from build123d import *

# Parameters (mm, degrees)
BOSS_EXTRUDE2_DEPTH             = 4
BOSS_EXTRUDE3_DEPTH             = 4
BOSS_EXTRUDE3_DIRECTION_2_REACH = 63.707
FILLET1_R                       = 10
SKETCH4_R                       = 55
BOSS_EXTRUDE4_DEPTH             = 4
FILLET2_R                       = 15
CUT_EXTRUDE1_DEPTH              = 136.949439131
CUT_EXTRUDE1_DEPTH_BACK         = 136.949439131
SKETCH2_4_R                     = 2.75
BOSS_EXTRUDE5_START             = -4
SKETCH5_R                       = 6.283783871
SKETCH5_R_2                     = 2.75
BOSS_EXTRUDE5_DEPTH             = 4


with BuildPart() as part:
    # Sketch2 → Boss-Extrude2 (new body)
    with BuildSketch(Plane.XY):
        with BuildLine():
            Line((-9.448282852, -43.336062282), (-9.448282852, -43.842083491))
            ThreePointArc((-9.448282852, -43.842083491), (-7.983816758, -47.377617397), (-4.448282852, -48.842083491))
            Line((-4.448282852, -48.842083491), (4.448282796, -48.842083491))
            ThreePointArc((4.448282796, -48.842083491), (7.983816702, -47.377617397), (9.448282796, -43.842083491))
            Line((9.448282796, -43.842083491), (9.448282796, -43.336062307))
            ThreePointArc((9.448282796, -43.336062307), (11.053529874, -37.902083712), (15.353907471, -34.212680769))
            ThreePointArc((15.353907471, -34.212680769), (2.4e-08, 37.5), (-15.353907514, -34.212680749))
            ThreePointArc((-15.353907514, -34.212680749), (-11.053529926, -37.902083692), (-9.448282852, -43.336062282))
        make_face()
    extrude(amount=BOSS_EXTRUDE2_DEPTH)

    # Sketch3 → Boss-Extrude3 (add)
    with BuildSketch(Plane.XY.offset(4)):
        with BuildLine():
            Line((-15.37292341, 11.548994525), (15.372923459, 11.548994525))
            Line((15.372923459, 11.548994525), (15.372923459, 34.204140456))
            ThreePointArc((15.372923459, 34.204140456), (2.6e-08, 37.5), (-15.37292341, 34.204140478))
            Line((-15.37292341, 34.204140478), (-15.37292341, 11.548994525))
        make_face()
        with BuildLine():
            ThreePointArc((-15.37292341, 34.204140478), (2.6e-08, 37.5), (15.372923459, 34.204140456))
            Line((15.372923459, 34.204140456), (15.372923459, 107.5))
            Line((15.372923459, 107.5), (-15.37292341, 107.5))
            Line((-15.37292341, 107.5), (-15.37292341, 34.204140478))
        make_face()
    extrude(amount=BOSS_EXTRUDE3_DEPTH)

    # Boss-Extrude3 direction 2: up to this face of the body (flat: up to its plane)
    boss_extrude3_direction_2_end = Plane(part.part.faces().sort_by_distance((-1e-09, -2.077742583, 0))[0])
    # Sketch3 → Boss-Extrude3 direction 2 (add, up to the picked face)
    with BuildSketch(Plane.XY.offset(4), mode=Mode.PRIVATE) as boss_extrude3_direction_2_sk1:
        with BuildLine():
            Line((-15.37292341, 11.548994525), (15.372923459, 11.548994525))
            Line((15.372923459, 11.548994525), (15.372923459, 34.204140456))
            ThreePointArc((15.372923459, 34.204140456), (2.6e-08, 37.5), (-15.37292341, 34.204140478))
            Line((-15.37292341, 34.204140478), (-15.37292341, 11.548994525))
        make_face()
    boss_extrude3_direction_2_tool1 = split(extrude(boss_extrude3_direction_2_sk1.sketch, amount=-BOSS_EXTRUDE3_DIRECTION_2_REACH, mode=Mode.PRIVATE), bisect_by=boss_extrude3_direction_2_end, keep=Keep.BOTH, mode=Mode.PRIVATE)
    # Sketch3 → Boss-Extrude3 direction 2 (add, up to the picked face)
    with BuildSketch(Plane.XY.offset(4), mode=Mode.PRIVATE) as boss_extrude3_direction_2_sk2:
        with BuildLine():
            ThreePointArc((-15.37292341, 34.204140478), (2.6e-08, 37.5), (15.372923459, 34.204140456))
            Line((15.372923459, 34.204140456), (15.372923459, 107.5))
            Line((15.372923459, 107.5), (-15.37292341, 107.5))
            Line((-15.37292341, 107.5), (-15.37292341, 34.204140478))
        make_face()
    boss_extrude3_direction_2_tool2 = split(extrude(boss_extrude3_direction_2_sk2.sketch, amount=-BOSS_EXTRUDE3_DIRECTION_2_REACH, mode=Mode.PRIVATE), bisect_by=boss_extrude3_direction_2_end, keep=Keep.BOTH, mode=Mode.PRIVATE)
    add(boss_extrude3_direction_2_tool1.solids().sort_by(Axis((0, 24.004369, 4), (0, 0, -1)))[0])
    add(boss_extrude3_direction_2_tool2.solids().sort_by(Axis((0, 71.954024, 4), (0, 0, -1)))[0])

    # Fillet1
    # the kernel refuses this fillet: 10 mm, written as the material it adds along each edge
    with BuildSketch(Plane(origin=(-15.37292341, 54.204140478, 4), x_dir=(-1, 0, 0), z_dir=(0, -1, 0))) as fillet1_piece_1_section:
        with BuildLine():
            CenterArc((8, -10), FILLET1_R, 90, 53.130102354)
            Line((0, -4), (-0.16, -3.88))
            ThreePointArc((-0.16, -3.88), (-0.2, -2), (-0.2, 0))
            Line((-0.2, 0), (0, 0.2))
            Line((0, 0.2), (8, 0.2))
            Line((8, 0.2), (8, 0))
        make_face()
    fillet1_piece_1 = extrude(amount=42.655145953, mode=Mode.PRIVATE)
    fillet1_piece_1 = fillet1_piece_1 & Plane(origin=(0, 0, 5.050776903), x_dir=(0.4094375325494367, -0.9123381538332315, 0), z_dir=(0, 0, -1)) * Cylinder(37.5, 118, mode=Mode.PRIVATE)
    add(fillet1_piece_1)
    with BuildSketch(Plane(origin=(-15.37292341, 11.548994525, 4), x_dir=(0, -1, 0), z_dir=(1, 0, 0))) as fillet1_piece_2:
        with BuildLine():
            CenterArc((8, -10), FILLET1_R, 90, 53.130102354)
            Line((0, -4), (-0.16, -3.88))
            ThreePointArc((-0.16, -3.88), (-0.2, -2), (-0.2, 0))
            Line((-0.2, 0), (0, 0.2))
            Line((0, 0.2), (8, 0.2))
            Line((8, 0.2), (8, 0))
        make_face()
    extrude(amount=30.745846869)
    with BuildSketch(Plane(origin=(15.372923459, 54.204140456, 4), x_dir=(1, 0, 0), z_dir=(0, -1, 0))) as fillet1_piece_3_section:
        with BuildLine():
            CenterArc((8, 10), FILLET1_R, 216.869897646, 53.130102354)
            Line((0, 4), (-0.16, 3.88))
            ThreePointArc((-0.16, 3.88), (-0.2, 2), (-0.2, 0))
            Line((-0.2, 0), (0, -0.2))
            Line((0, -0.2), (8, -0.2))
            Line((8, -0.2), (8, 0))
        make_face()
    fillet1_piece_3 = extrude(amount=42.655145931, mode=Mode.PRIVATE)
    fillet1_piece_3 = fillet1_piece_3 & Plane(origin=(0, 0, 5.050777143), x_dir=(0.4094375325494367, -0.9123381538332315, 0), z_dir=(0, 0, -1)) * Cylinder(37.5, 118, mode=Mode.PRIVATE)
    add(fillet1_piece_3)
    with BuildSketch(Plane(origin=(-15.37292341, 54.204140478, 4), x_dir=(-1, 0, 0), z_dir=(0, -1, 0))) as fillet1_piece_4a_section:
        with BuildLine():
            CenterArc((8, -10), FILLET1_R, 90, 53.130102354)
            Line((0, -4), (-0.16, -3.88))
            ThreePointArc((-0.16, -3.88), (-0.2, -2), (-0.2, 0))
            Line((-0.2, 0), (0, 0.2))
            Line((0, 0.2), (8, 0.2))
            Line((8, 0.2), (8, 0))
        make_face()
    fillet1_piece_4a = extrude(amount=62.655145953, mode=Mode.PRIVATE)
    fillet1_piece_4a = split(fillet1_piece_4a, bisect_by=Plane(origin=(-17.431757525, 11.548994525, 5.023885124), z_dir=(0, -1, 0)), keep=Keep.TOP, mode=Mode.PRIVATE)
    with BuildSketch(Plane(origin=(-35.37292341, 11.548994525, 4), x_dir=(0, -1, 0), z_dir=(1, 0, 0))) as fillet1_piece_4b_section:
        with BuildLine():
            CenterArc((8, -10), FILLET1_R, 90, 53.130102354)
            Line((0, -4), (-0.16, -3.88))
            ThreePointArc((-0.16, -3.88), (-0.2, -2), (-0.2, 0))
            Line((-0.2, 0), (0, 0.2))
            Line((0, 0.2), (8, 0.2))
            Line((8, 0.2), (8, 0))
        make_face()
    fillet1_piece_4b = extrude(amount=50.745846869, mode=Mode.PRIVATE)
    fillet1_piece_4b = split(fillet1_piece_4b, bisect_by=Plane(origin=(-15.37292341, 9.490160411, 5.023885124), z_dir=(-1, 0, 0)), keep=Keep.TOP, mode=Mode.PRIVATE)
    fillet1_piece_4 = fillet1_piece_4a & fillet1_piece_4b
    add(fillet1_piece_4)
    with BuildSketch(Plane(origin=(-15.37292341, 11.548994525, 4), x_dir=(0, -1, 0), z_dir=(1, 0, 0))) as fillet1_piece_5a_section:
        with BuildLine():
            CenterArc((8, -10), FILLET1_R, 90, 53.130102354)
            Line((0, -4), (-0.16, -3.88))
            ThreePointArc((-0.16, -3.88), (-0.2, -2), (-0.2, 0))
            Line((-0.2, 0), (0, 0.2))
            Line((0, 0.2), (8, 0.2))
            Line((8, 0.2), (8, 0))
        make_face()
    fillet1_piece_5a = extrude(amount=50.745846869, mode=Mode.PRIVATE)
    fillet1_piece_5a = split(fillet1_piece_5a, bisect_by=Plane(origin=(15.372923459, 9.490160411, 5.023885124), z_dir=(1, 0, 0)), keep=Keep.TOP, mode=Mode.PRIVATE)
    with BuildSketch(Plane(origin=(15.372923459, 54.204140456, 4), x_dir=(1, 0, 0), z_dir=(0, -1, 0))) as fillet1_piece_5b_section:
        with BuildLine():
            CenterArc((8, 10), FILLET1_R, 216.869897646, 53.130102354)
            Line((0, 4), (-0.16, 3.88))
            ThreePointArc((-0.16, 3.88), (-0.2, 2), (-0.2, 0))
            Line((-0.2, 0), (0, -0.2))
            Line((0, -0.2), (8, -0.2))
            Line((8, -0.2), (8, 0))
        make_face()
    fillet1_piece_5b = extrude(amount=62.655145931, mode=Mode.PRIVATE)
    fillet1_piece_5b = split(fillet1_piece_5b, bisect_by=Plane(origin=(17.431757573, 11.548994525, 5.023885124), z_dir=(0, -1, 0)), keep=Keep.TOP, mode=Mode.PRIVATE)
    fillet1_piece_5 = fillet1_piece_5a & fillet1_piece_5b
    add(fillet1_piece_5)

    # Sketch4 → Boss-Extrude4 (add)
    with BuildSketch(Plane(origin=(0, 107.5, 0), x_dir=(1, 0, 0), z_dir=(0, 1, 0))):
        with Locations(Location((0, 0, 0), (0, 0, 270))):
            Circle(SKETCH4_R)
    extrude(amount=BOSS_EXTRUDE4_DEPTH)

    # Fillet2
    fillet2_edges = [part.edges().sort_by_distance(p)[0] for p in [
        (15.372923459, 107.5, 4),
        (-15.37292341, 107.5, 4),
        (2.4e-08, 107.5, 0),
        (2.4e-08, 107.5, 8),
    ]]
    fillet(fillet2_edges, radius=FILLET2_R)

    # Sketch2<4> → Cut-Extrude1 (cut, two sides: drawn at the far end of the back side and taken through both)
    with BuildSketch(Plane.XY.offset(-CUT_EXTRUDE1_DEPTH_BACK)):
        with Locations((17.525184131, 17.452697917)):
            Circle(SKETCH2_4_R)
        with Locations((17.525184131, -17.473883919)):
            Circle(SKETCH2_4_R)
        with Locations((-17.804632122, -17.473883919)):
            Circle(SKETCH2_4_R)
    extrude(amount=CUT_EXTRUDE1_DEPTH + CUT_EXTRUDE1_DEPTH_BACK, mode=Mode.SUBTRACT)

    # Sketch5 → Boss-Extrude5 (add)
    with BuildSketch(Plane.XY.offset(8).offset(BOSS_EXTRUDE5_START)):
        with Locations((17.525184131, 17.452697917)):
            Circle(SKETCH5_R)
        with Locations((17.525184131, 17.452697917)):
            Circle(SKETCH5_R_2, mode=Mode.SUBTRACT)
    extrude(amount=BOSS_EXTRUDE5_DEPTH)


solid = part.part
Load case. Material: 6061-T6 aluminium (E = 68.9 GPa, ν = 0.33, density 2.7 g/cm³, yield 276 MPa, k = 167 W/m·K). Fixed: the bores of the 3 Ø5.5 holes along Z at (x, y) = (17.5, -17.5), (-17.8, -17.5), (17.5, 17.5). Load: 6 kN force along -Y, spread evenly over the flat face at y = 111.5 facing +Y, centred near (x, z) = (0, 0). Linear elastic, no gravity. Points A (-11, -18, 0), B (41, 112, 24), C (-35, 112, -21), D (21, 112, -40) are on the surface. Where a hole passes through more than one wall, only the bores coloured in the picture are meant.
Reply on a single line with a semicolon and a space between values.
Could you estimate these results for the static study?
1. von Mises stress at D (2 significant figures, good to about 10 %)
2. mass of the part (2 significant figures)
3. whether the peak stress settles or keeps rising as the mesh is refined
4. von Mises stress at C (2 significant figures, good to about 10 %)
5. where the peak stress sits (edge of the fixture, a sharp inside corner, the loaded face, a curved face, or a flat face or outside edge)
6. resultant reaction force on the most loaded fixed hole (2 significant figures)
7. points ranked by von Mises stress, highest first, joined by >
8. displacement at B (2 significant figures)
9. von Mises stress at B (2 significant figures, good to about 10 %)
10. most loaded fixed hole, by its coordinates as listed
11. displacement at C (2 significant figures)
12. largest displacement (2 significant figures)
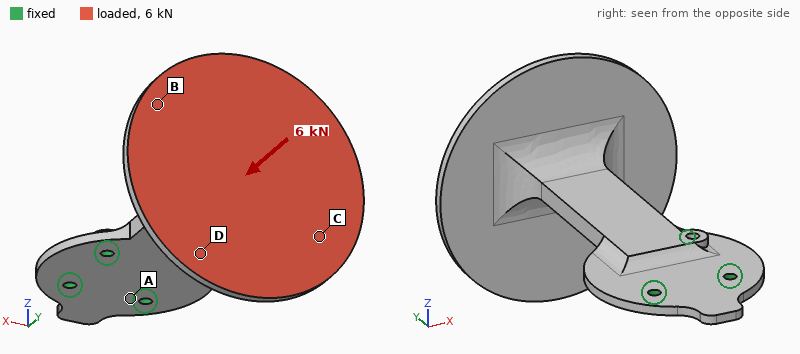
28 MPa; 220 g; keeps rising; 68 MPa; edge of the fixture; 2.8 kN; C > B > D > A; 1.2 mm; 47 MPa; (17.5, 17.5); 1.5 mm; 2.4 mm
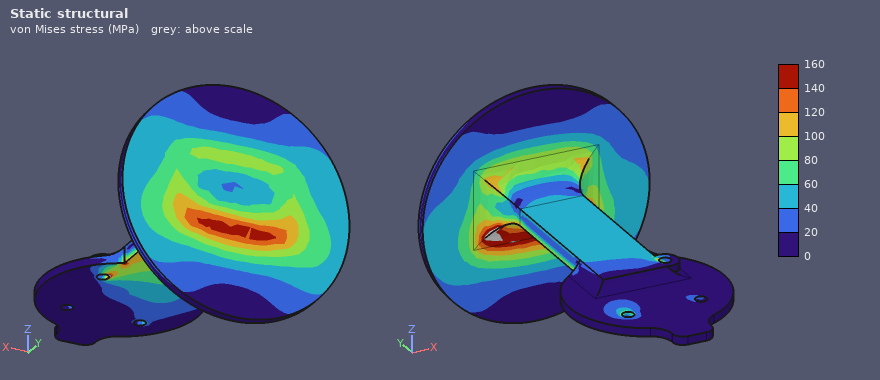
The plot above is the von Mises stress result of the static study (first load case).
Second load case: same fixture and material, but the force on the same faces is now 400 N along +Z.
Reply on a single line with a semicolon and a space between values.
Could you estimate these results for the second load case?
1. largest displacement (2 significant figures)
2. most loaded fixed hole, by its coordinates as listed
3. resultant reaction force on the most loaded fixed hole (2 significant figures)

1.9 mm; (17.5, 17.5); 1.0 kN
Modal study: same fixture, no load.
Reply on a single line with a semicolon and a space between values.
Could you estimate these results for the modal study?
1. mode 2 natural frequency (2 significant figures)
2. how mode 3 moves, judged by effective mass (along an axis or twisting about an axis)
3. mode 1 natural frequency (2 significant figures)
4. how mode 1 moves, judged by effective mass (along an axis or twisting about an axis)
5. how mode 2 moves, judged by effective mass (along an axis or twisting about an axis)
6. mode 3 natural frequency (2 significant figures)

460 Hz; along X; 230 Hz; along Z; twisting about Y; 930 Hz
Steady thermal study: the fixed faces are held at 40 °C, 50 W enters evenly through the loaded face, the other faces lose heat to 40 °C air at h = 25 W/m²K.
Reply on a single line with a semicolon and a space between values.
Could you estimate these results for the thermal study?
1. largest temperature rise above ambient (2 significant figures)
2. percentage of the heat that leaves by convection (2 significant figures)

70 K; 47 %
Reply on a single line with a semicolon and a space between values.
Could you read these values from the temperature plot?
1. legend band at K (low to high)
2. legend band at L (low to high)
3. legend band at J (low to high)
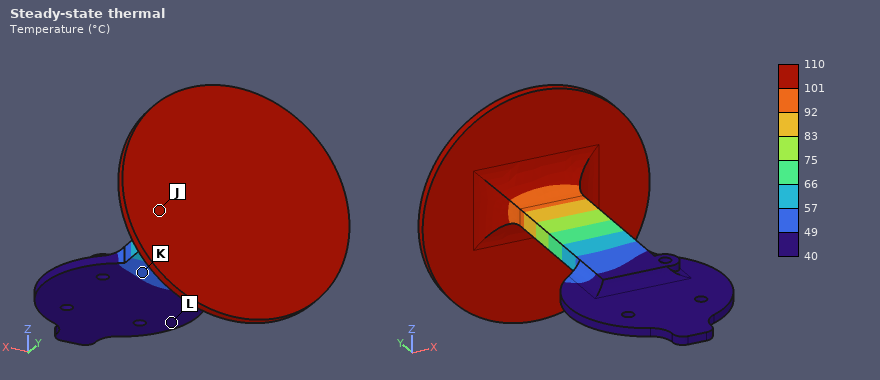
49 to 57 °C; 40 to 49 °C; 101 to 110 °C
